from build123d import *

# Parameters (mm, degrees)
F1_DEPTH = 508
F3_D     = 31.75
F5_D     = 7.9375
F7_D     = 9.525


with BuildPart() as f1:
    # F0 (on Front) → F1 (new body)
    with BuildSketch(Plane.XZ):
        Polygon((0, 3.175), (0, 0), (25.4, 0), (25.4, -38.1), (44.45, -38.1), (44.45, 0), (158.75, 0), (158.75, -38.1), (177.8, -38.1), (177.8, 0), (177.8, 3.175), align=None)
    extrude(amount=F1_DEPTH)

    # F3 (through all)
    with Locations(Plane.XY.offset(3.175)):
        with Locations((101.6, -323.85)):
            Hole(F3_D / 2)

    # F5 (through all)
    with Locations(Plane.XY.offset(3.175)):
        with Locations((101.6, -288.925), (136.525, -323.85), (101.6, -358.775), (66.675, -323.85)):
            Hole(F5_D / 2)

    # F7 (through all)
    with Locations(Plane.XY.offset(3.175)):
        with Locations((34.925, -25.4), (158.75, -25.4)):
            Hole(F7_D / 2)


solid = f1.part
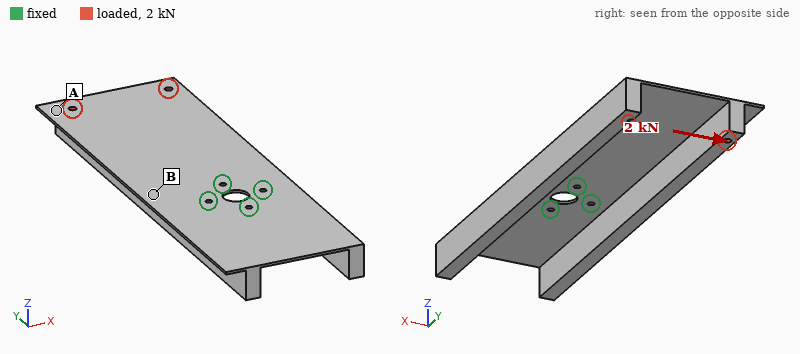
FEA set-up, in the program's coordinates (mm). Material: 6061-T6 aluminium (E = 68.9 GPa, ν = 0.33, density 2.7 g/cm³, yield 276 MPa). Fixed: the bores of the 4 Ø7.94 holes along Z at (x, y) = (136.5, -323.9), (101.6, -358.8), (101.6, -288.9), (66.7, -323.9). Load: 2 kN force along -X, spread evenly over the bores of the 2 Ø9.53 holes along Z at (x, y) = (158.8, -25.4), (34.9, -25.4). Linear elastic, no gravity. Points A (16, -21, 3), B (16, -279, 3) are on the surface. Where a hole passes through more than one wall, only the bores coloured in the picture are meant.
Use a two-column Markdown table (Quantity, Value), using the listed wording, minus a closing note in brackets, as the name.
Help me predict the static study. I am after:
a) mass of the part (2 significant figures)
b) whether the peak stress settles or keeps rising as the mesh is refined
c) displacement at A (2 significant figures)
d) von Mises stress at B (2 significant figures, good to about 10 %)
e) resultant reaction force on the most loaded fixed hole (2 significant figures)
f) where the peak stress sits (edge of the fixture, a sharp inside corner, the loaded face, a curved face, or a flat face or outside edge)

| Quantity | Value |
|---|---|
| mass of the part | 2.7 kg |
| whether the peak stress settles or keeps rising as the mesh is refined | keeps rising |
| displacement at A | 0.91 mm |
| von Mises stress at B | 14 MPa |
| resultant reaction force on the most loaded fixed hole | 4.7 kN |
| where the peak stress sits | edge of the fixture |
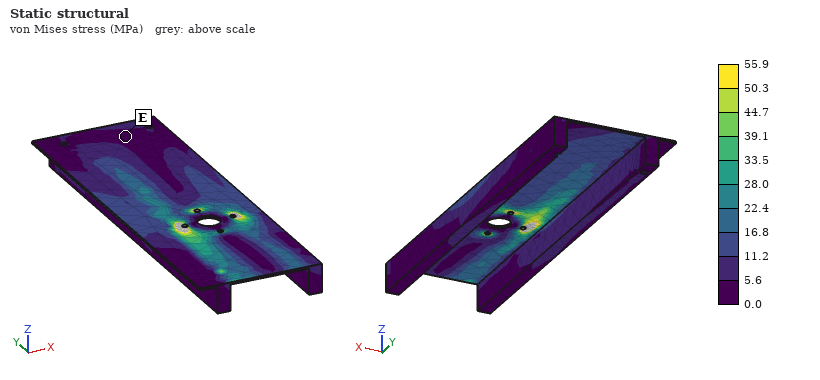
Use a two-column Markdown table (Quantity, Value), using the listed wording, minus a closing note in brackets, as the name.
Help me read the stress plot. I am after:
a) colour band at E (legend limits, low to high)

| Quantity | Value |
|---|---|
| colour band at E | 0.0 to 5.6 MPa |
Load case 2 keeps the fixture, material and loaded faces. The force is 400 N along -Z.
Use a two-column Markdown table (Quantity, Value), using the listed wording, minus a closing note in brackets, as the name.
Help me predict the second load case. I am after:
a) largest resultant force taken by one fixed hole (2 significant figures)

| Quantity | Value |
|---|---|
| largest resultant force taken by one fixed hole | 1.0 kN |
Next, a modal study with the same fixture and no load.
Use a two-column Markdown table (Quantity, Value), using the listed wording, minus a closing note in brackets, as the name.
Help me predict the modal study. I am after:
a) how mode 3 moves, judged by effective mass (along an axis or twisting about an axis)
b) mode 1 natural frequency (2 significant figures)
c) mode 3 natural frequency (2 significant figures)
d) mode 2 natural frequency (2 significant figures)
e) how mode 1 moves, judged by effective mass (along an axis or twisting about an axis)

| Quantity | Value |
|---|---|
| how mode 3 moves, judged by effective mass | along Z |
| mode 1 natural frequency | 59 Hz |
| mode 3 natural frequency | 220 Hz |
| mode 2 natural frequency | 140 Hz |
| how mode 1 moves, judged by effective mass | along Z |
